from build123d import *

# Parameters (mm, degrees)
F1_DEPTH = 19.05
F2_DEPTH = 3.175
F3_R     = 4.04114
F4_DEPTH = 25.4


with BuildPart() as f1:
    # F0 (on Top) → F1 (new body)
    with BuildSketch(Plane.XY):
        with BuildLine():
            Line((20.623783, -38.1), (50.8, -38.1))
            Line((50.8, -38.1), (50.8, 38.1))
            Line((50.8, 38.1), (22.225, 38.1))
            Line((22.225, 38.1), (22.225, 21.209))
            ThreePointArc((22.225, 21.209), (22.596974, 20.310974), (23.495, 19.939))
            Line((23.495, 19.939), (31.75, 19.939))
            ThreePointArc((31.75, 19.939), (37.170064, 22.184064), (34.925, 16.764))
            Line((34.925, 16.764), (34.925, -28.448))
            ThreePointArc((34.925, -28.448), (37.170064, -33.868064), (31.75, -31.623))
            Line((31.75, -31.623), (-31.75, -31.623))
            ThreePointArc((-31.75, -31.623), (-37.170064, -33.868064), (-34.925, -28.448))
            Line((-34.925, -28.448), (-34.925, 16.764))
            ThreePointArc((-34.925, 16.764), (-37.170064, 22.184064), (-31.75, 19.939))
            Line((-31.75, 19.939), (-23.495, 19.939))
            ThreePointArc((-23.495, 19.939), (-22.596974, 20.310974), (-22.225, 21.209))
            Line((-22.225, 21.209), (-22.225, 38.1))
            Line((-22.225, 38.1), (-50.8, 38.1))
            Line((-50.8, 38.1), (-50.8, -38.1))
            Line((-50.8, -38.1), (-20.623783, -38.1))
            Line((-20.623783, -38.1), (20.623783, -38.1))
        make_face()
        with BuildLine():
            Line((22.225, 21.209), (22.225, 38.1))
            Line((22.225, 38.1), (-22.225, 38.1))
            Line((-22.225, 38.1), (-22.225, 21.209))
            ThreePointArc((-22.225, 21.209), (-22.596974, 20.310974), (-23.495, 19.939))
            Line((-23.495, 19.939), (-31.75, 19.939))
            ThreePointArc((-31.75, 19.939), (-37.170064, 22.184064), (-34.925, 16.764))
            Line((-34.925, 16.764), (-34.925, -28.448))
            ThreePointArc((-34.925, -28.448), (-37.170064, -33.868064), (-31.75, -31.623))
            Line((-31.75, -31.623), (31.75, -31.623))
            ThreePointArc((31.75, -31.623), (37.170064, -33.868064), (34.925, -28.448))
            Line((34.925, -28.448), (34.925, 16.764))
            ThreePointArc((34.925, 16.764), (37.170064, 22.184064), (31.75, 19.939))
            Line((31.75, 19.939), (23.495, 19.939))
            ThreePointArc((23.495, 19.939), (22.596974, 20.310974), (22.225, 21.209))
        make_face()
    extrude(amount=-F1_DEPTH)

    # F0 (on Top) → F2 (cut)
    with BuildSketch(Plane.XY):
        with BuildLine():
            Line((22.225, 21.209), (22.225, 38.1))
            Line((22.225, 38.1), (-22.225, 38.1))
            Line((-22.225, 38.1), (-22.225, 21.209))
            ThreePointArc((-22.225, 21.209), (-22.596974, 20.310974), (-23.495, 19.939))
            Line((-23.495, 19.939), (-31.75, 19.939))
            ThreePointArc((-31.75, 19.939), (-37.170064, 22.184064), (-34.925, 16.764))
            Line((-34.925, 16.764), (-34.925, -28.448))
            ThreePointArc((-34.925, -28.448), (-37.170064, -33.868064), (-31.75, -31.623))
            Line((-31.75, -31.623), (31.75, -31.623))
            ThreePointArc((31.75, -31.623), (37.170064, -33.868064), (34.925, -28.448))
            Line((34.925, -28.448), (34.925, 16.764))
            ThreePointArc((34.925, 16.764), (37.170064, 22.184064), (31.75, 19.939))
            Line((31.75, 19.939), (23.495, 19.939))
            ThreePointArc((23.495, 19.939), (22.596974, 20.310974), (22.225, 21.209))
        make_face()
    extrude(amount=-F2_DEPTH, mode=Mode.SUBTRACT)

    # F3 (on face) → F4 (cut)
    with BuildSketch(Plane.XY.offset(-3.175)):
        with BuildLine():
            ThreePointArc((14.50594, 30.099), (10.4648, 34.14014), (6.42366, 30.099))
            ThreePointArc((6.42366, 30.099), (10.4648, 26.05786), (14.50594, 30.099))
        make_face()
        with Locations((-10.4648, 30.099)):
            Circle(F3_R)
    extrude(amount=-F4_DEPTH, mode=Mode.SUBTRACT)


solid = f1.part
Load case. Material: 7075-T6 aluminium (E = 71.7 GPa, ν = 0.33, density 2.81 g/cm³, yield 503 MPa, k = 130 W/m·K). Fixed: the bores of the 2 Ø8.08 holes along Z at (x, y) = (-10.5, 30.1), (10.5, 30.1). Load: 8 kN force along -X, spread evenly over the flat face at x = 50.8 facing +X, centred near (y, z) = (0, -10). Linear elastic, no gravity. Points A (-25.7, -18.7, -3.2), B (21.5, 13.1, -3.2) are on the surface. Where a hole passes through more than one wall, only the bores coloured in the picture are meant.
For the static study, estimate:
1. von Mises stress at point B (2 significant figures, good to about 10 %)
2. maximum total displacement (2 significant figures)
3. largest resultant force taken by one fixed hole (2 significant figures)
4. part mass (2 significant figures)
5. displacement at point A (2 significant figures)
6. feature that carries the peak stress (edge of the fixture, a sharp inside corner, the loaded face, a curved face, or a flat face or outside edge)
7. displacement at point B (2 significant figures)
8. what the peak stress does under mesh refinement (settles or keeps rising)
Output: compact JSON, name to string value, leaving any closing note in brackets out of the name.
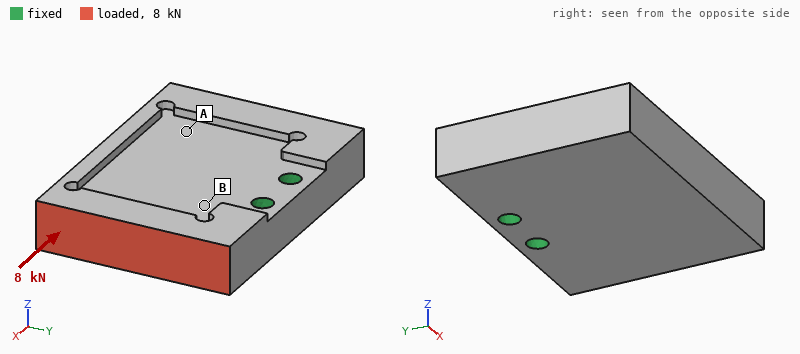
{"von Mises stress at point B": "16 MPa", "maximum total displacement": "63 µm", "largest resultant force taken by one fixed hole": "9.3 kN", "part mass": "370 g", "displacement at point A": "37 µm", "feature that carries the peak stress": "edge of the fixture", "displacement at point B": "18 µm", "what the peak stress does under mesh refinement": "keeps rising"}
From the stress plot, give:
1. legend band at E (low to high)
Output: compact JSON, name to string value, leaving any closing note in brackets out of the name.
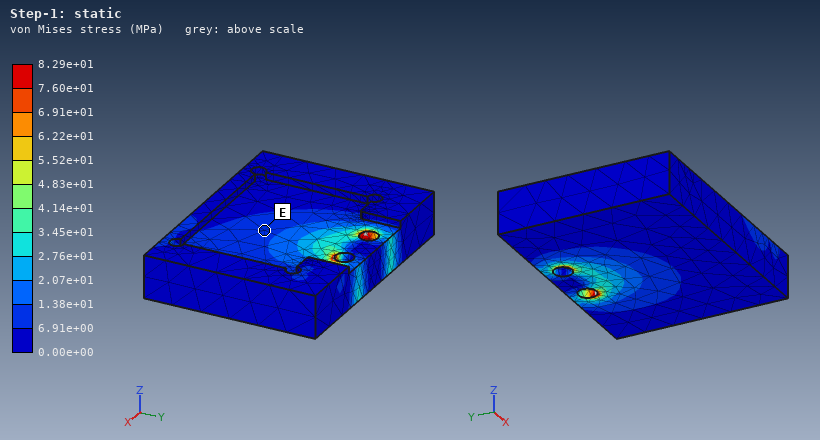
{"legend band at E": "6.91e+00 to 1.38e+01 MPa"}
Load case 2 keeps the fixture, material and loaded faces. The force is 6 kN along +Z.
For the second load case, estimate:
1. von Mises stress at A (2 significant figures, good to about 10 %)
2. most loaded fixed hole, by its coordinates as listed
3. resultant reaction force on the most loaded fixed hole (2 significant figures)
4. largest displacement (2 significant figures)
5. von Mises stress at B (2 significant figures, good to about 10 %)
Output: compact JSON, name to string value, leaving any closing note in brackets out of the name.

{"von Mises stress at A": "23 MPa", "most loaded fixed hole, by its coordinates as listed": "(10.5, 30.1)", "resultant reaction force on the most loaded fixed hole": "8.7 kN", "largest displacement": "0.34 mm", "von Mises stress at B": "61 MPa"}
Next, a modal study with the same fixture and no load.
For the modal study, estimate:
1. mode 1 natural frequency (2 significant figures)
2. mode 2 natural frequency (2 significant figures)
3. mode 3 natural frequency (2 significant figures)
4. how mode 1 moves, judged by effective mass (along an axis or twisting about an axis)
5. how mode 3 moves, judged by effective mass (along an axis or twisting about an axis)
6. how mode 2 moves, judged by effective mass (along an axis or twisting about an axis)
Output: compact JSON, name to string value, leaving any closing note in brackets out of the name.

{"mode 1 natural frequency": "2100 Hz", "mode 2 natural frequency": "3000 Hz", "mode 3 natural frequency": "3400 Hz", "how mode 1 moves, judged by effective mass": "along Z", "how mode 3 moves, judged by effective mass": "along X", "how mode 2 moves, judged by effective mass": "twisting about Y"}
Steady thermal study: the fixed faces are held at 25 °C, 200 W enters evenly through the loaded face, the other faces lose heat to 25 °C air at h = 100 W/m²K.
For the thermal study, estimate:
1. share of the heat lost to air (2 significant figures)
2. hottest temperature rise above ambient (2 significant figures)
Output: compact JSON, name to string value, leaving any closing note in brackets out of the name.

{"share of the heat lost to air": "25 %", "hottest temperature rise above ambient": "67 K"}
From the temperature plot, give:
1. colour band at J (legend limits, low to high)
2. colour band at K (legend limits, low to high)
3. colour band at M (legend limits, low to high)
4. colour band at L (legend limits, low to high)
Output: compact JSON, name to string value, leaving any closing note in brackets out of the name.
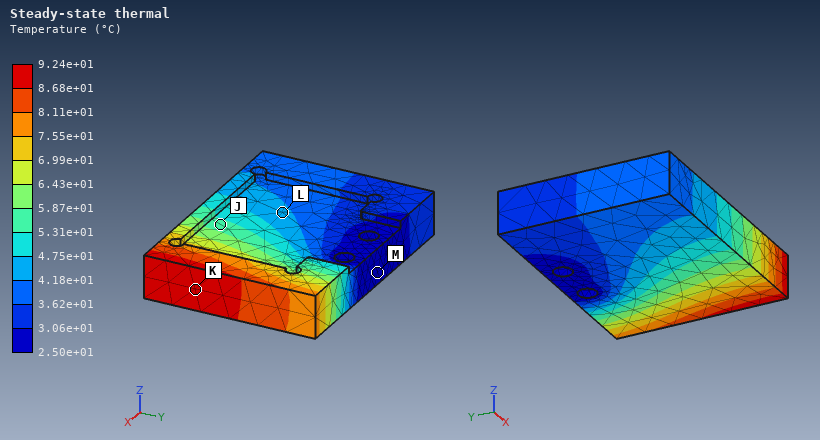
{"colour band at J": "5.31e+01 to 5.87e+01 °C", "colour band at K": "8.68e+01 to 9.24e+01 °C", "colour band at M": "2.50e+01 to 3.06e+01 °C", "colour band at L": "4.18e+01 to 4.75e+01 °C"}
